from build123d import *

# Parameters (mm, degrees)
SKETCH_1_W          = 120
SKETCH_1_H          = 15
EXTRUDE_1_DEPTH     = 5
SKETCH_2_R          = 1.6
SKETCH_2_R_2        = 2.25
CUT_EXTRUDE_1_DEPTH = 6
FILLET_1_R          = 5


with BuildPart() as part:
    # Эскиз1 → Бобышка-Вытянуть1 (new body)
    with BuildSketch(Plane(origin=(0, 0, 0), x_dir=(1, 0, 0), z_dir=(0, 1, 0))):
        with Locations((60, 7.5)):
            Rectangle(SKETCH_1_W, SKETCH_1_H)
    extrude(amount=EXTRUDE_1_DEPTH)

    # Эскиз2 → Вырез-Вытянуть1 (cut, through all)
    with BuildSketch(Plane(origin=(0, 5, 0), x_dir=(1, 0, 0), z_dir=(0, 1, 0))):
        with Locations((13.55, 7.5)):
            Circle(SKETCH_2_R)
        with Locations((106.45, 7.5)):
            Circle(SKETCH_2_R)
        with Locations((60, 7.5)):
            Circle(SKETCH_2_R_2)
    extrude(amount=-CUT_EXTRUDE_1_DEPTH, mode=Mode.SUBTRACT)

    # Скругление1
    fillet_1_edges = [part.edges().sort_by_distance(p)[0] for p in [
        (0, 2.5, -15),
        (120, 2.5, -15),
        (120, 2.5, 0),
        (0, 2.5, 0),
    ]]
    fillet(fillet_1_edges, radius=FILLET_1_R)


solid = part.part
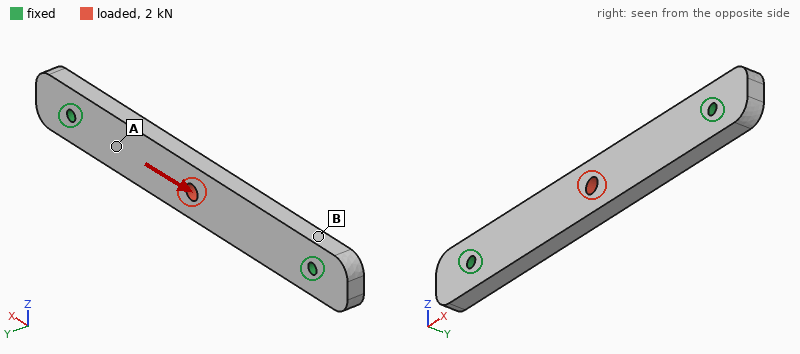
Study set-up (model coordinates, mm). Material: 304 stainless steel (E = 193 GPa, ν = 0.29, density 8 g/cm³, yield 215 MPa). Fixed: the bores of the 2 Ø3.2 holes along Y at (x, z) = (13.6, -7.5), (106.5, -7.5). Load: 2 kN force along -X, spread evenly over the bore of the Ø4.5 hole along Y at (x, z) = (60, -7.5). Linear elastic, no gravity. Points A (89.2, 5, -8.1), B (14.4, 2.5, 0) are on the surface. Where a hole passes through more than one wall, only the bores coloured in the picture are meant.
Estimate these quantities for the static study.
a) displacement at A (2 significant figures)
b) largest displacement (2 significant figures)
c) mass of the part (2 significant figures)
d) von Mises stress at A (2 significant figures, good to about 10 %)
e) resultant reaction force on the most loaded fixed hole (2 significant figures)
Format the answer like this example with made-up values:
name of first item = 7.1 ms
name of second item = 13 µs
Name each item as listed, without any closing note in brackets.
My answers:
displacement at A = 1.4 µm
largest displacement = 3.7 µm
mass of the part = 70 g
von Mises stress at A = 13 MPa
resultant reaction force on the most loaded fixed hole = 1.0 kN
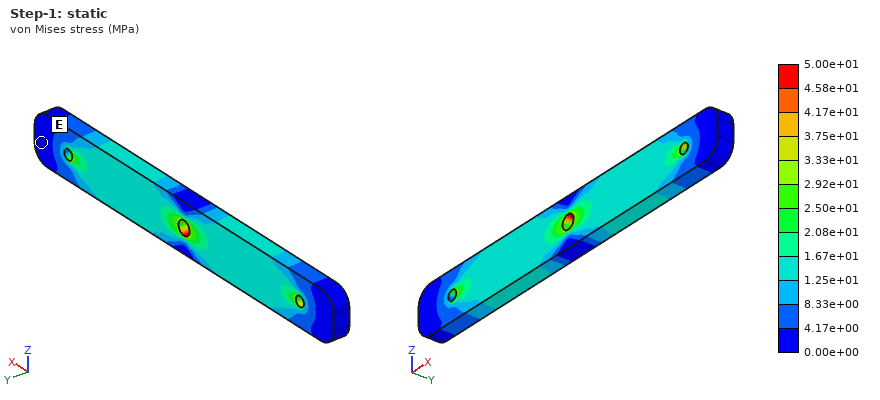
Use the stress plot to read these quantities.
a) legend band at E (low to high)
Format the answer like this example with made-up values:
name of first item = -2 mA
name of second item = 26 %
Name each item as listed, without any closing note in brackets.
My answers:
legend band at E = 0.00e+00 to 4.17e+00 MPa
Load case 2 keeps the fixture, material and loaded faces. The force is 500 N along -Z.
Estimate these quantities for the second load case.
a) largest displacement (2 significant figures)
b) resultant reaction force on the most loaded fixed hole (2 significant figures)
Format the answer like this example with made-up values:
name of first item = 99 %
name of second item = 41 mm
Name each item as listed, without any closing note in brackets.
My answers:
largest displacement = 17 µm
resultant reaction force on the most loaded fixed hole = 250 N
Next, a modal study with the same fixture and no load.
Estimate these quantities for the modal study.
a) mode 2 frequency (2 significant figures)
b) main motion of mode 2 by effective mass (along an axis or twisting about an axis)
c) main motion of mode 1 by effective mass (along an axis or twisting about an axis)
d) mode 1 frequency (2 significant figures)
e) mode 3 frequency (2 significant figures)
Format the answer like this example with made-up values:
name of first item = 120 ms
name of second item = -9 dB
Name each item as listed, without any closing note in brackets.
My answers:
mode 2 frequency = 5500 Hz
main motion of mode 2 by effective mass = along Z
main motion of mode 1 by effective mass = along Y
mode 1 frequency = 2800 Hz
mode 3 frequency = 7600 Hz
